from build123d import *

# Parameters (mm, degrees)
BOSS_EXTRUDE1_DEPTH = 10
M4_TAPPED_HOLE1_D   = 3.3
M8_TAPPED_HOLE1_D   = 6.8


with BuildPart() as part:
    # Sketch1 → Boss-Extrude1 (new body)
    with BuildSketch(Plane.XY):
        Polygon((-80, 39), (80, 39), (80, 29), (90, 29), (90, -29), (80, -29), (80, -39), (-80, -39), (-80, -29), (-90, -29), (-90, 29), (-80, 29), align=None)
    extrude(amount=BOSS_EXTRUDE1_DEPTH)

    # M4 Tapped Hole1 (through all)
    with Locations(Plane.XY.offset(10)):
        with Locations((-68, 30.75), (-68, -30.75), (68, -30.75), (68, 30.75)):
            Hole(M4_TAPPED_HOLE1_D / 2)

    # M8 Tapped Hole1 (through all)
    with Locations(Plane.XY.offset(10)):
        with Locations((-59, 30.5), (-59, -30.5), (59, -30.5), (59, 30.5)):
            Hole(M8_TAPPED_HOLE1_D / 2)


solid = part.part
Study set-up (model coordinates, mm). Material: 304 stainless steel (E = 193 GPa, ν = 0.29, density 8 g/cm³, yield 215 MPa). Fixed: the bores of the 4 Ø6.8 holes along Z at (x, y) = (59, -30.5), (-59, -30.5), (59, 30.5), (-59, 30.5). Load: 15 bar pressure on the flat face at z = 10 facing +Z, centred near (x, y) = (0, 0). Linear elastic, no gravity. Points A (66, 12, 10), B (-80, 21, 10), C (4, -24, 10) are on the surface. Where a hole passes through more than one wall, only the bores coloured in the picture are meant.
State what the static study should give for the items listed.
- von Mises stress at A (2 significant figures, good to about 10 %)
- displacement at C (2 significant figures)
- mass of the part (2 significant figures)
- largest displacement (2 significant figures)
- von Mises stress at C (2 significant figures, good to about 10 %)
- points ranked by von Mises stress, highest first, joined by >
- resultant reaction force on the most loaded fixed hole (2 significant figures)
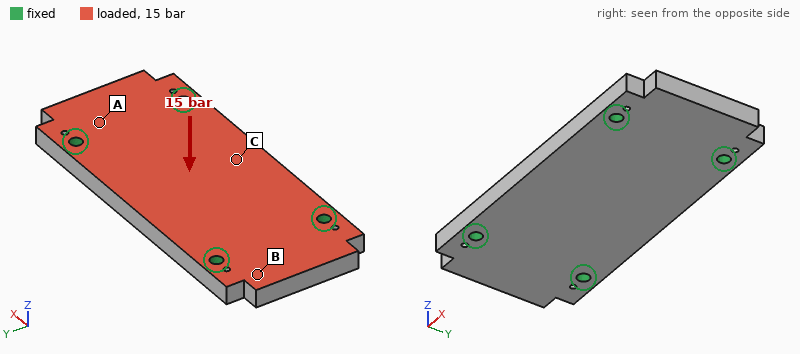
33 MPa
57 µm
1.1 kg
58 µm
51 MPa
C > A > B
5.0 kN
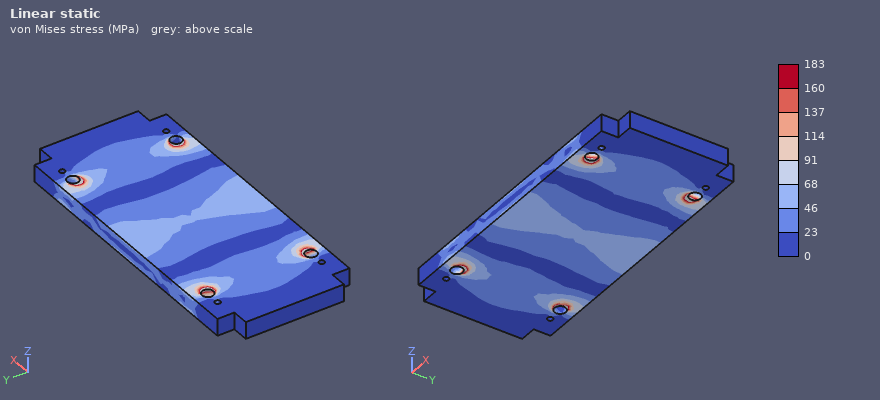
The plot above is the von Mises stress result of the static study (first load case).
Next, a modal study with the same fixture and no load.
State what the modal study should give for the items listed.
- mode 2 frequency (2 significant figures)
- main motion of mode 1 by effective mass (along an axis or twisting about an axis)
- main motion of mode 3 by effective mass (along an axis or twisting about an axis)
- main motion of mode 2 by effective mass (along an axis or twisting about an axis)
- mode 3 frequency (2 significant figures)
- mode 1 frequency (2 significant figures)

4900 Hz
along Z
twisting about Y
twisting about X
6200 Hz
3100 Hz
